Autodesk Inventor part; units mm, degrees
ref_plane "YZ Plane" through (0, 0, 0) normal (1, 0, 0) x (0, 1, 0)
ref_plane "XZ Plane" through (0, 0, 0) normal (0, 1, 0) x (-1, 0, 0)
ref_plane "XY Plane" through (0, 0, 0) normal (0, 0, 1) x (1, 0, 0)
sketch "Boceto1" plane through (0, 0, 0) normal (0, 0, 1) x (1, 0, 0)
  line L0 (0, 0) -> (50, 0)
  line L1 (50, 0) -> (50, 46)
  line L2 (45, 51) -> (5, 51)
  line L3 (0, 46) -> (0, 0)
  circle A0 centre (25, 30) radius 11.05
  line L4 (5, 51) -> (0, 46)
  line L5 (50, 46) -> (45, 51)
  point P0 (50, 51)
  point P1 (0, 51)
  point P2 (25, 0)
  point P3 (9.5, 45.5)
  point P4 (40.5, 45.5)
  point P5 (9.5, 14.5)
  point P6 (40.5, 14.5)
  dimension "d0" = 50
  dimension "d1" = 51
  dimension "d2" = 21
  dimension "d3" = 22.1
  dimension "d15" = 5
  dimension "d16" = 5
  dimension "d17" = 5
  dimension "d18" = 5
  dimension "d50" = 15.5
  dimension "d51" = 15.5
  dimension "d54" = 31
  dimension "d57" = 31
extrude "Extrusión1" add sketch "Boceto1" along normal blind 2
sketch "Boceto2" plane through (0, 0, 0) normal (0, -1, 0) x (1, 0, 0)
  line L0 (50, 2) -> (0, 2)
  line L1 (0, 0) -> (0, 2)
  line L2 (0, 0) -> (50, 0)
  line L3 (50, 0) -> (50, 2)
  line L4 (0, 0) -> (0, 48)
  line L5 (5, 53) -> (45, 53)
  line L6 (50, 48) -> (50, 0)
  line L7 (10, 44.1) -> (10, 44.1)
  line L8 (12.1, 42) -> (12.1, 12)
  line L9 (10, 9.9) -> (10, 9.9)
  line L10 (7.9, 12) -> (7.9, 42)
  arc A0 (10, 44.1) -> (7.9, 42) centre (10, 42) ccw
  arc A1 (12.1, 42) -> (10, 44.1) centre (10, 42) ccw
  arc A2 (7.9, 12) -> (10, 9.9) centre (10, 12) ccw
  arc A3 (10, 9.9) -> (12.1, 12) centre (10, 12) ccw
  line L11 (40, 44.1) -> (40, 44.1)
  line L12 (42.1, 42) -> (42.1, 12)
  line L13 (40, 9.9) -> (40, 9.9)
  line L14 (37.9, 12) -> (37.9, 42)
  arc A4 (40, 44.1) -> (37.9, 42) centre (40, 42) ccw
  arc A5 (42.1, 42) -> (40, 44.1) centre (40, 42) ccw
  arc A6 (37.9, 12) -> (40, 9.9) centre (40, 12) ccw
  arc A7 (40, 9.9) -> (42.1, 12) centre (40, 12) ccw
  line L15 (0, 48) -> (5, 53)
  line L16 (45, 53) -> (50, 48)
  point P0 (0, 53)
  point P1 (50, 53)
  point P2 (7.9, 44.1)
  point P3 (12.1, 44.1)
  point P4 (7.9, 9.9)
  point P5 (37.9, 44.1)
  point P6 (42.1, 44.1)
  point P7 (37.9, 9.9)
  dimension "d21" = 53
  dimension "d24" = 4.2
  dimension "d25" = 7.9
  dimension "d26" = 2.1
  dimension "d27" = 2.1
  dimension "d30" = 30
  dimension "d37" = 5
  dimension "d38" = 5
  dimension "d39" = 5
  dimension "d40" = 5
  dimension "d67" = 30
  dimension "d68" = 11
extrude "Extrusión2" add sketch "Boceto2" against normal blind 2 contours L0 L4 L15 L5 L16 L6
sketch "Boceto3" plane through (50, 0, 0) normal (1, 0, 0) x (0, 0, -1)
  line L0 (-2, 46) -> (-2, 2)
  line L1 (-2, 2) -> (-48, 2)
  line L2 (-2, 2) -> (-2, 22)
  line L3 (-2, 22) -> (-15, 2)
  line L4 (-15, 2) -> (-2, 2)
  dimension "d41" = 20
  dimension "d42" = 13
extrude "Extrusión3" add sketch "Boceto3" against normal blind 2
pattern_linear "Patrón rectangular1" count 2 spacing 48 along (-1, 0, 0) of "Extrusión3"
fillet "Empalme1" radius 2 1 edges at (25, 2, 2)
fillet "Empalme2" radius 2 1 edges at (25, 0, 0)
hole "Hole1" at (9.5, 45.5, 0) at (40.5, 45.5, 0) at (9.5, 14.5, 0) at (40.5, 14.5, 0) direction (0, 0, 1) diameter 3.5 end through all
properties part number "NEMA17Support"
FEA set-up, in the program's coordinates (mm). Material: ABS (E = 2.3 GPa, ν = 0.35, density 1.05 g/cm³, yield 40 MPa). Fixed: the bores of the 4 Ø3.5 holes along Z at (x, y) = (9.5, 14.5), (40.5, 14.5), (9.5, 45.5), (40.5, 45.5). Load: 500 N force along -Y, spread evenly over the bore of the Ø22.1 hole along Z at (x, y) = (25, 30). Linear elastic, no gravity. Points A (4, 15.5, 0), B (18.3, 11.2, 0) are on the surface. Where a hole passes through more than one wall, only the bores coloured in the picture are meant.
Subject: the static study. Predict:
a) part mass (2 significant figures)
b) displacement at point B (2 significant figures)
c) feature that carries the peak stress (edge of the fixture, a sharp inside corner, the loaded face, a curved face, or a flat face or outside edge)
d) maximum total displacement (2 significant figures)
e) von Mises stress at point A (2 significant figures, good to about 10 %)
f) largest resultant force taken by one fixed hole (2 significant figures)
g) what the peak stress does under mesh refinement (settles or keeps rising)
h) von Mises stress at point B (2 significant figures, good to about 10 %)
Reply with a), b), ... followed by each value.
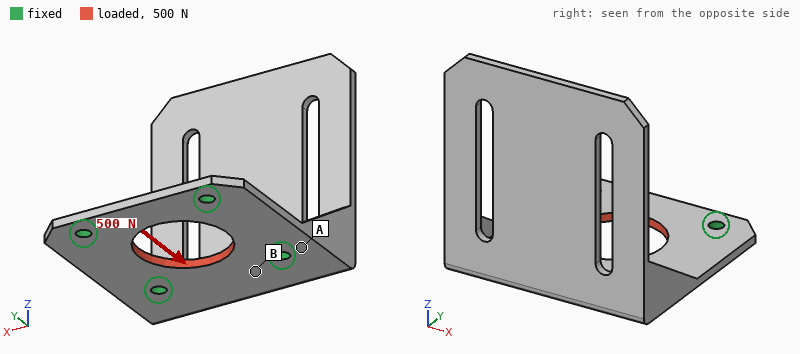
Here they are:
a) 9.7 g
b) 23 µm
c) edge of the fixture
d) 69 µm
e) 0.91 MPa
f) 130 N
g) keeps rising
h) 2.7 MPa
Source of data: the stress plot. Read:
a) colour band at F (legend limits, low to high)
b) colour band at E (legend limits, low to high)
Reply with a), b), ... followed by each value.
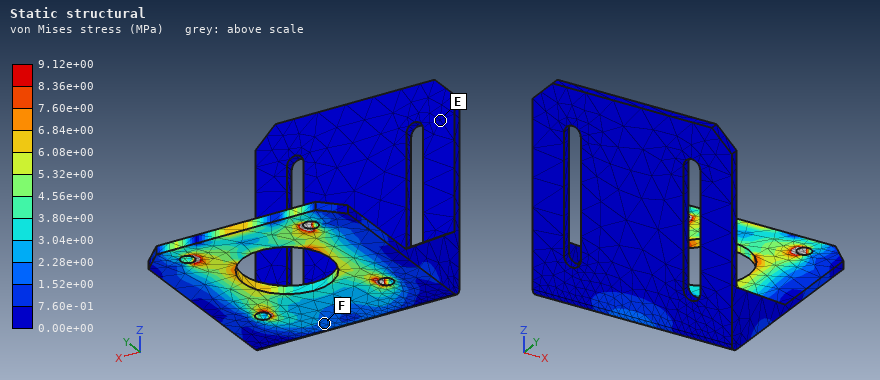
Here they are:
a) 1.52e+00 to 2.28e+00 MPa
b) 0.00e+00 to 7.60e-01 MPa
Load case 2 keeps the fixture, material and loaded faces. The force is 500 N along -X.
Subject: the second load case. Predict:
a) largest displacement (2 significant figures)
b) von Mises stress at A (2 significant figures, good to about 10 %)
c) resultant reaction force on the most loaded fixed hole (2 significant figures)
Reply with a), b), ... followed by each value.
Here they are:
a) 52 µm
b) 2.2 MPa
c) 130 N
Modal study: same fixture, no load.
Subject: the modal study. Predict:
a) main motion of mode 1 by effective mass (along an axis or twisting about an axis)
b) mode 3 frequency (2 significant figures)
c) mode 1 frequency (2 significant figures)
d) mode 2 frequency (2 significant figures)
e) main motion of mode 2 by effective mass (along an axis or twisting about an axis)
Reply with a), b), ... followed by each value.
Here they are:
a) along Y
b) 650 Hz
c) 190 Hz
d) 430 Hz
e) along X
